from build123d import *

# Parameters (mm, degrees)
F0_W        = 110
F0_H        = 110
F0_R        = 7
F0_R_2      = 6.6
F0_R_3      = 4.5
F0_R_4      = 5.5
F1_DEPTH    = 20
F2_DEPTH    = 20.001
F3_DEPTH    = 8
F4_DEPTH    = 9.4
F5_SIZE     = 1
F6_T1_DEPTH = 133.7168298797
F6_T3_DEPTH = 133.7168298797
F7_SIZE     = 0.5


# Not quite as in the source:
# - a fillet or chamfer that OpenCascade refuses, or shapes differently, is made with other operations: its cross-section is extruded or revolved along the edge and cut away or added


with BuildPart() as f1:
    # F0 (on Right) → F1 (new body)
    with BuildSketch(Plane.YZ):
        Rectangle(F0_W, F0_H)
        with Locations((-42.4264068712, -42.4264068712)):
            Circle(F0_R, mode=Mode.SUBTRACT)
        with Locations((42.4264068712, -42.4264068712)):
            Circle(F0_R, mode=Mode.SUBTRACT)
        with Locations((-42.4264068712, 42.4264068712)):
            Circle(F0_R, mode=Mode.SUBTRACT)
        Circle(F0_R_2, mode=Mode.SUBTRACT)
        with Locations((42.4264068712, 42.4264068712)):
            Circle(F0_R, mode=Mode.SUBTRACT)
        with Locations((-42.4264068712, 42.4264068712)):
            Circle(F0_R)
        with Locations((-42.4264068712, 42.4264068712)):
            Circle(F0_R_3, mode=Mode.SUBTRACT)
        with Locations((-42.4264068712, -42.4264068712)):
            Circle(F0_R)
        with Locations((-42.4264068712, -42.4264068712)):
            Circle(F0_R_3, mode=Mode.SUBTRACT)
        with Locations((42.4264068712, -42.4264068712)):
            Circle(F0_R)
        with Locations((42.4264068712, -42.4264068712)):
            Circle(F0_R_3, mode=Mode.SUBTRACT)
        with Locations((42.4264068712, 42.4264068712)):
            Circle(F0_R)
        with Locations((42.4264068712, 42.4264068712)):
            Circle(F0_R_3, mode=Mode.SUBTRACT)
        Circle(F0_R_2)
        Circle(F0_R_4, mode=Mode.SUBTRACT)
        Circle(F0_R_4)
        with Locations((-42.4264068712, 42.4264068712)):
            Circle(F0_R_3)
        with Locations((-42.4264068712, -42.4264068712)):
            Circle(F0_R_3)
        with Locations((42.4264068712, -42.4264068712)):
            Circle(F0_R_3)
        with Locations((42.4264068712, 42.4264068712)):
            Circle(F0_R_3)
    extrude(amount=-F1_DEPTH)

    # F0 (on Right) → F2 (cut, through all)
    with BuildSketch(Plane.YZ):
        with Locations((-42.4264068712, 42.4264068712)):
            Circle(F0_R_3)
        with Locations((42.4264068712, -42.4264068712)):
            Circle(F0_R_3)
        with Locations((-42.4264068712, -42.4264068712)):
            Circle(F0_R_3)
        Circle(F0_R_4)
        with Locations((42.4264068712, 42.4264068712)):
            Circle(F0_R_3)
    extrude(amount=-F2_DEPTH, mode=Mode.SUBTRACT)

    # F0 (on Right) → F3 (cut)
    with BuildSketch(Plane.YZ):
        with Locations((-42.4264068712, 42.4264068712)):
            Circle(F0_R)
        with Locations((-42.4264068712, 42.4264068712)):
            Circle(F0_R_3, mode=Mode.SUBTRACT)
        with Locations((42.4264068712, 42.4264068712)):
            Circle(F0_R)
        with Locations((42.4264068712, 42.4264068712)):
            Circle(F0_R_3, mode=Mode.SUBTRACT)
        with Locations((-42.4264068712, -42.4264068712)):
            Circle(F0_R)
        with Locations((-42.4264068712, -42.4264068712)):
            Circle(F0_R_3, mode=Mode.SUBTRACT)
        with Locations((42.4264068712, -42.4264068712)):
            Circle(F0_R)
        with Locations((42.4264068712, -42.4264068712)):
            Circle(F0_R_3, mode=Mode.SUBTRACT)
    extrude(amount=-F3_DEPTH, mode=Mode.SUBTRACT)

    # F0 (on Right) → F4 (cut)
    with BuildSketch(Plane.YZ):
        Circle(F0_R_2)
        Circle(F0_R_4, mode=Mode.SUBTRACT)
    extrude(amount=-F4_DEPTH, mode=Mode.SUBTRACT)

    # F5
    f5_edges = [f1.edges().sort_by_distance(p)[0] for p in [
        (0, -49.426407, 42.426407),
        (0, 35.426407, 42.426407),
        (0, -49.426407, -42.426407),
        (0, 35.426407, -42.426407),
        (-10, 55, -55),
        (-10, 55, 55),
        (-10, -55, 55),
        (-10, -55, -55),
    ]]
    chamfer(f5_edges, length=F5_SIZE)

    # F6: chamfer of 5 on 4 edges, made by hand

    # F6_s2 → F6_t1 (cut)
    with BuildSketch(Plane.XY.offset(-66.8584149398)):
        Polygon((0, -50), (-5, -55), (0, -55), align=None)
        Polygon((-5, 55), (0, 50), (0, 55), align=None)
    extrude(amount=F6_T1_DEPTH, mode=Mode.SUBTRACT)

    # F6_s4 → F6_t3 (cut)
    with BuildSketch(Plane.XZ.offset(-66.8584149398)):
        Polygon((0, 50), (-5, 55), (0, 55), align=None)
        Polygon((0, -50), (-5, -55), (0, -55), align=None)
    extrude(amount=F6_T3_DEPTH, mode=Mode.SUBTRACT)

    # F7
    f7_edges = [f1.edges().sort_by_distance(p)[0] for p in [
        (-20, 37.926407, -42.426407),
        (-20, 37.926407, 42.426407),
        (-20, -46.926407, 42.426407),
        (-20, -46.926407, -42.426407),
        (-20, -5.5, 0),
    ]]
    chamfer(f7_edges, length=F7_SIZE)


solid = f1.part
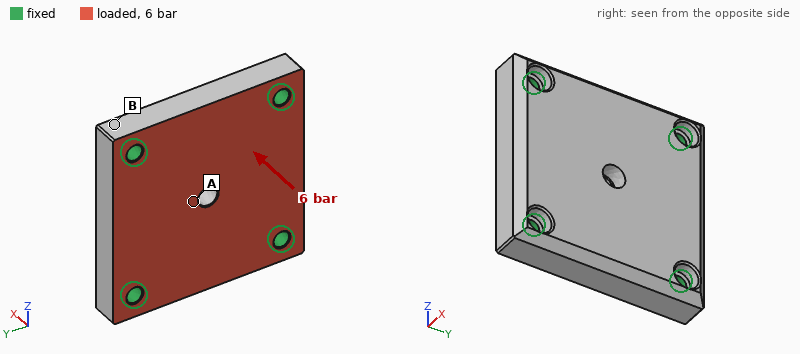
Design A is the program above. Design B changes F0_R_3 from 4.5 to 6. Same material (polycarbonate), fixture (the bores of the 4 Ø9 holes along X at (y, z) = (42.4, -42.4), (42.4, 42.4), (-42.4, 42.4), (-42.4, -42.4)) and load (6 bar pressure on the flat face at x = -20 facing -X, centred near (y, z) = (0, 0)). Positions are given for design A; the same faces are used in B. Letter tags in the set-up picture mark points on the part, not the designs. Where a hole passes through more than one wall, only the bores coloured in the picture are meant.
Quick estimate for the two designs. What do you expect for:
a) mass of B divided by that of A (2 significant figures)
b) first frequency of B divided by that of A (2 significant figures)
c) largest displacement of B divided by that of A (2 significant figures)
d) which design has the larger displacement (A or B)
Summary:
0.99
1.1
0.85
A
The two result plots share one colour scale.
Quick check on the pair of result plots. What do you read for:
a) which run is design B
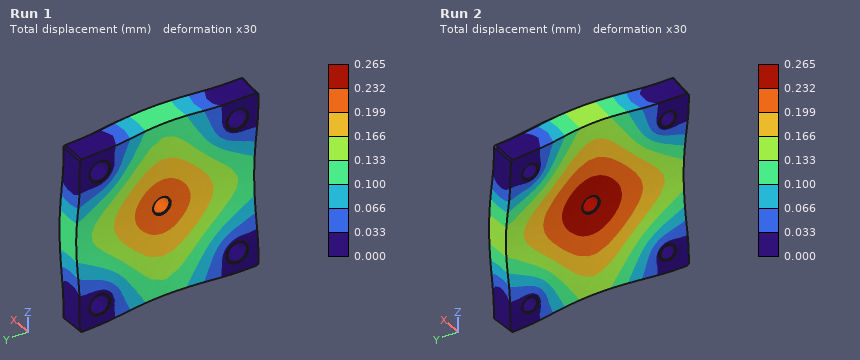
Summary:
Run 1
